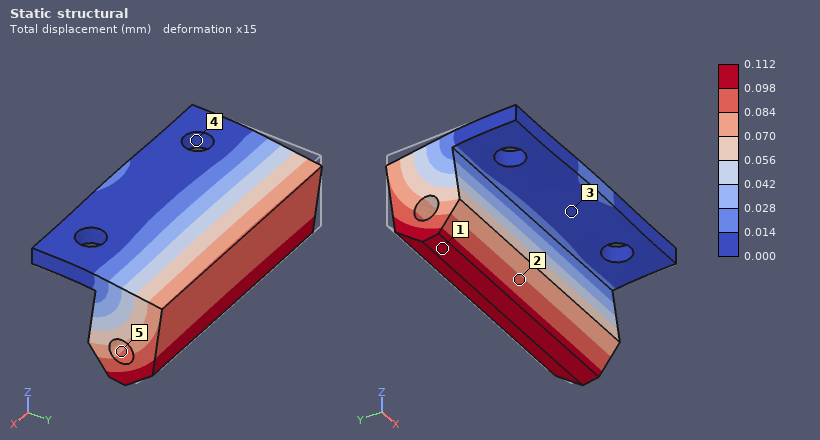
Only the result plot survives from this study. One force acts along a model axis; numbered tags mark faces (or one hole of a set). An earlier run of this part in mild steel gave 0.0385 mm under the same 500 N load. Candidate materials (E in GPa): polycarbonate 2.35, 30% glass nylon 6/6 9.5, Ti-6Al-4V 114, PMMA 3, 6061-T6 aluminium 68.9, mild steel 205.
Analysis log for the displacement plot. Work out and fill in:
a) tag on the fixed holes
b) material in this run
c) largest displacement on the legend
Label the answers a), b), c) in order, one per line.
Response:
a) 4
b) 6061-T6 aluminium
c) 0.112 mm
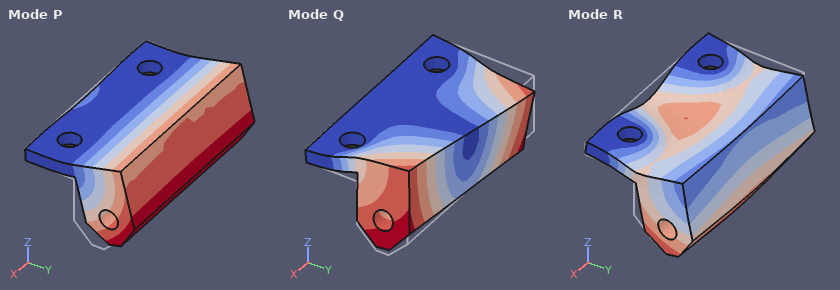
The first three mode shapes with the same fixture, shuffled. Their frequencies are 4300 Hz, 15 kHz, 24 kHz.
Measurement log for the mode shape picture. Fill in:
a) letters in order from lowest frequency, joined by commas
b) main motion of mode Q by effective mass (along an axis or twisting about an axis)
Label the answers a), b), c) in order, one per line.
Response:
a) P, Q, R
b) along X
